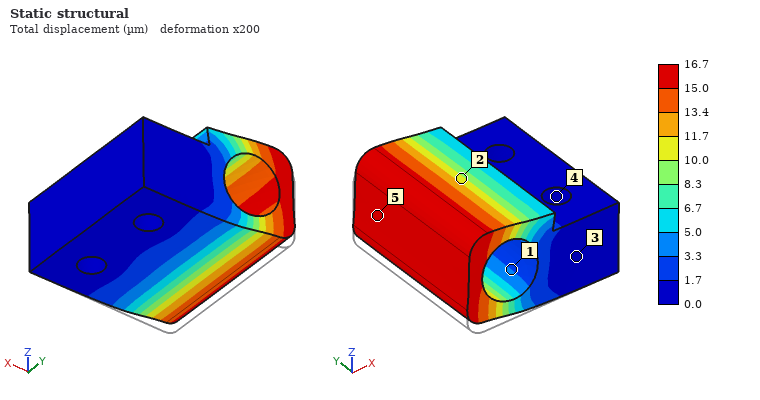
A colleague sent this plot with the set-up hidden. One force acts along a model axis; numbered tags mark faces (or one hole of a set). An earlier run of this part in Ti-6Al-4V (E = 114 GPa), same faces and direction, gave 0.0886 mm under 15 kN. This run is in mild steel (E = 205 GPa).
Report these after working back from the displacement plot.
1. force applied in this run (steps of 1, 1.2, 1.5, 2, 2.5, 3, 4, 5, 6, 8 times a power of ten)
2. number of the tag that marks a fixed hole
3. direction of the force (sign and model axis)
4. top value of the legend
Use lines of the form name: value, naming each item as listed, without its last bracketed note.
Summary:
force applied in this run: 5 kN
number of the tag that marks a fixed hole: 4
direction of the force: +Z
top value of the legend: 16.7 µm
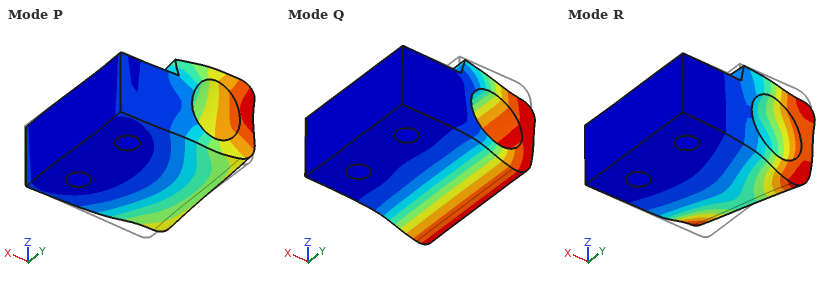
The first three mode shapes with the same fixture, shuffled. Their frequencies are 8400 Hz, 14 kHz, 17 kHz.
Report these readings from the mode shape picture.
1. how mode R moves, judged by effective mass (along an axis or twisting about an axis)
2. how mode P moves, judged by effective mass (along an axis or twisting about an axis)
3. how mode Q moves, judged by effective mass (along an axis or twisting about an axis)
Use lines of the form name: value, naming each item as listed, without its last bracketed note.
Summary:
how mode R moves, judged by effective mass: twisting about X
how mode P moves, judged by effective mass: along Y
how mode Q moves, judged by effective mass: along Z
